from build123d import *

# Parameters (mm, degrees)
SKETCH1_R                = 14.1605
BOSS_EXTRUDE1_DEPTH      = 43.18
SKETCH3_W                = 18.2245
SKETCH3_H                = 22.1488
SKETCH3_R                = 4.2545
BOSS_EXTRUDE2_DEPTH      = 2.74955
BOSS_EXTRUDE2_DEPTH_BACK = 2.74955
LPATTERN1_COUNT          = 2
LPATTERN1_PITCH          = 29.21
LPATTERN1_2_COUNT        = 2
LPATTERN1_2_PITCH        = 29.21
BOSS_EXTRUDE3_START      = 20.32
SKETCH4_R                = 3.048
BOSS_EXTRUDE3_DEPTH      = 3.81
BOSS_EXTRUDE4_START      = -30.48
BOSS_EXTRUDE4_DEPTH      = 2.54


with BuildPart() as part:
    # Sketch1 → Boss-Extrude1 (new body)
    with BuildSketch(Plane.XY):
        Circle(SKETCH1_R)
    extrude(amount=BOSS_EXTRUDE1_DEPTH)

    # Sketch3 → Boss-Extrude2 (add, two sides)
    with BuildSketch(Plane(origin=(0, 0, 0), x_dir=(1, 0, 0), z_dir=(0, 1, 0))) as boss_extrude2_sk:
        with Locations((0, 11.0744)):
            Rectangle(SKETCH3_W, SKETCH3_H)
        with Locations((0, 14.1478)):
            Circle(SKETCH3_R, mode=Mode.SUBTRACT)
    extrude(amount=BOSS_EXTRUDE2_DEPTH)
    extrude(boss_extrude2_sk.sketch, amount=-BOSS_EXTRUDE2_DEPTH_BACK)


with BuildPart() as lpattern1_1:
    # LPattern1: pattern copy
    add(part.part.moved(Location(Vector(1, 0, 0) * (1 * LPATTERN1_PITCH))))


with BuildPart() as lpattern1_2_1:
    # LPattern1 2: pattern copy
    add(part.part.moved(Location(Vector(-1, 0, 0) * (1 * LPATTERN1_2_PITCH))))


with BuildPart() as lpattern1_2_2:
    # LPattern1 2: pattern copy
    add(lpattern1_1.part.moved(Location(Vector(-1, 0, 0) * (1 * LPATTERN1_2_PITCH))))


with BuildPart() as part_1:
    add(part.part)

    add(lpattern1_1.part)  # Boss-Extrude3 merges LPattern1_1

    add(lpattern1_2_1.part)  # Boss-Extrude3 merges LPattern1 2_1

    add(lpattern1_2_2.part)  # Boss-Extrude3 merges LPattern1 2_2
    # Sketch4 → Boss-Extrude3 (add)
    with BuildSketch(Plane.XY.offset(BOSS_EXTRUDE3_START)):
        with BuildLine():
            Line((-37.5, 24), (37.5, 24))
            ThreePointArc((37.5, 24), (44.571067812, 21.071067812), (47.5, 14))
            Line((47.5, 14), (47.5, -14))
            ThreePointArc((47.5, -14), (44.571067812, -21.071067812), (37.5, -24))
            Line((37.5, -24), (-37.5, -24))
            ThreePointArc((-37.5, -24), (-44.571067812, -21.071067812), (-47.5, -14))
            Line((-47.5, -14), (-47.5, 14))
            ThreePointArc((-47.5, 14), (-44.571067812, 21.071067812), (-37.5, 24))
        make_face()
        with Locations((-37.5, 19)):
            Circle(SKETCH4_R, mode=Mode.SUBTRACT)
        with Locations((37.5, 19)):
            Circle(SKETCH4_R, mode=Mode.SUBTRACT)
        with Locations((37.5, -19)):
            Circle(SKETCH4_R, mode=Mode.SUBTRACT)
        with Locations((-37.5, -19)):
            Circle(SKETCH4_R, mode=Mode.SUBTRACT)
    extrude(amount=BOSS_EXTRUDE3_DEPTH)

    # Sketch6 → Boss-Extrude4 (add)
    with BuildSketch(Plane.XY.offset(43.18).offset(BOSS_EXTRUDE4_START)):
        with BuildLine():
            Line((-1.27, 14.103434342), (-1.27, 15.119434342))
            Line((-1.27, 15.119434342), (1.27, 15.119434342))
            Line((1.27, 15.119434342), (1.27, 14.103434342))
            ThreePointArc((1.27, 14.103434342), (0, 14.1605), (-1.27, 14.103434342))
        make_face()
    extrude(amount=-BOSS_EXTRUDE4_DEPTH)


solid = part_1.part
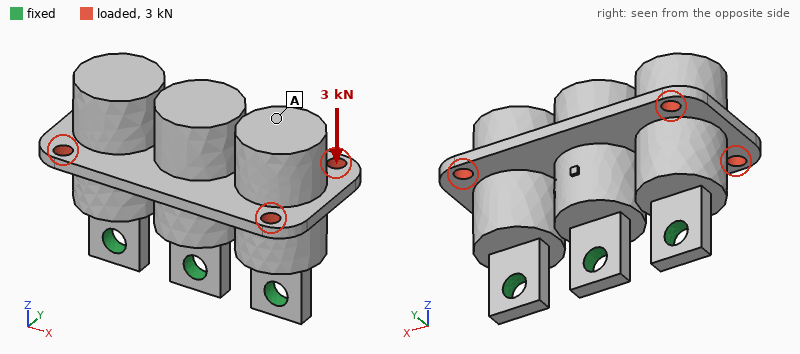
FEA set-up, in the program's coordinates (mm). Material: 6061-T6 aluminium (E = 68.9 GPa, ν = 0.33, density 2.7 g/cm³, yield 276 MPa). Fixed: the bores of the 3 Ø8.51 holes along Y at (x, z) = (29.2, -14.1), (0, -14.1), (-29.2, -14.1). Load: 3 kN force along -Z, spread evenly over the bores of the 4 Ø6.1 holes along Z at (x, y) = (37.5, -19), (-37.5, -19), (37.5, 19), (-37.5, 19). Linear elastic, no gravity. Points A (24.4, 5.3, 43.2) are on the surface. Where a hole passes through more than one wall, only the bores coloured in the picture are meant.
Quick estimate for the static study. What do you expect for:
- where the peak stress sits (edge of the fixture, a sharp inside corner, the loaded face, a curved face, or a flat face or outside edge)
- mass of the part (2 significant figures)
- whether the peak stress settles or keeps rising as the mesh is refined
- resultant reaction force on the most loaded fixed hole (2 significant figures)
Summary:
a sharp inside corner
260 g
keeps rising
1.5 kN
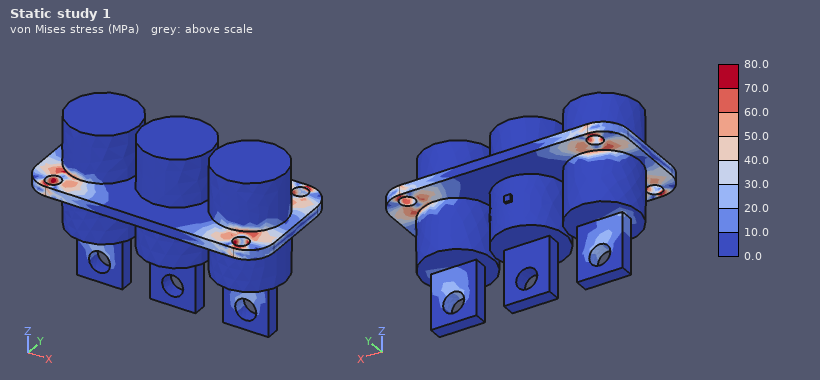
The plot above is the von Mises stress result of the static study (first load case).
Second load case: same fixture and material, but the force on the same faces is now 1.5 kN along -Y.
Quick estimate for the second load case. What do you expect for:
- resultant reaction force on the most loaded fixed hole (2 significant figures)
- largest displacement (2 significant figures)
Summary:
520 N
0.49 mm
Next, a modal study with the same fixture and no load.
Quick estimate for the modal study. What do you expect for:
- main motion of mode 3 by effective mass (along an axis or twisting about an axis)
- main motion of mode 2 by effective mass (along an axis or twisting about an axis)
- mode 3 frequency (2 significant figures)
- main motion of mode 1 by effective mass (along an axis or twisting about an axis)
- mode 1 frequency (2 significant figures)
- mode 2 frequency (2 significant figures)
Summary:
along X
twisting about Z
3900 Hz
along Y
690 Hz
1900 Hz
